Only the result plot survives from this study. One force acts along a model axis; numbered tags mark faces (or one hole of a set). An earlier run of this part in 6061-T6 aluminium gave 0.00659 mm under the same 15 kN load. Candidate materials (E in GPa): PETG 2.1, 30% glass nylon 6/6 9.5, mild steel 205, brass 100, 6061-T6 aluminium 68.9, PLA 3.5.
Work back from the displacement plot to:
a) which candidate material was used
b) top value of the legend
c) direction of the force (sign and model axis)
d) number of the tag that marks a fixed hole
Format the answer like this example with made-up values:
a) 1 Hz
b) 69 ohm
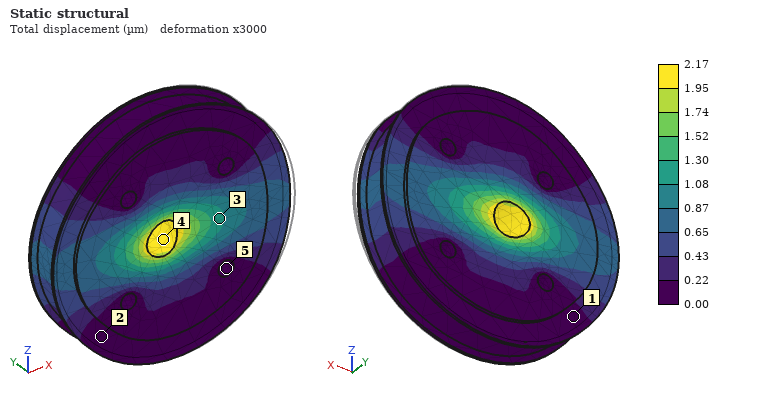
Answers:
a) mild steel
b) 2.17 µm
c) -X
d) 5
